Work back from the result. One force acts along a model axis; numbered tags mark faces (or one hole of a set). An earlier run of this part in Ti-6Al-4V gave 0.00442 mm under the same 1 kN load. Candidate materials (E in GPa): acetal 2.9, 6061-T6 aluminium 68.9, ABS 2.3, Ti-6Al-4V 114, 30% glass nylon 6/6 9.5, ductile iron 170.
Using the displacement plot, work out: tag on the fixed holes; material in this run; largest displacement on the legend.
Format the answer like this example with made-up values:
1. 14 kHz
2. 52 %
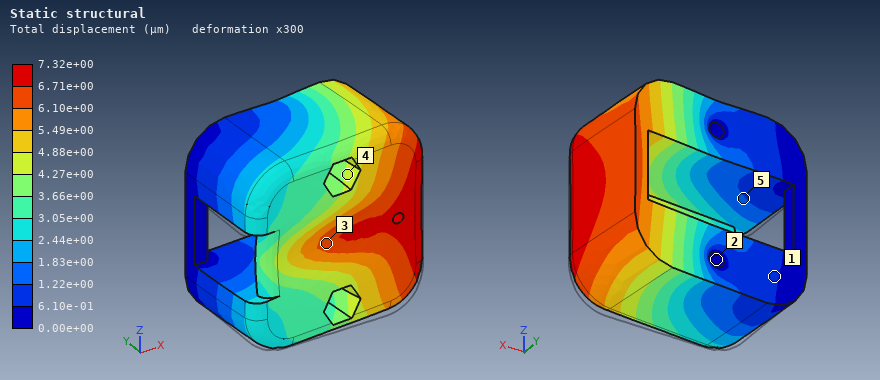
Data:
1. 2
2. 6061-T6 aluminium
3. 7.32e+00 µm
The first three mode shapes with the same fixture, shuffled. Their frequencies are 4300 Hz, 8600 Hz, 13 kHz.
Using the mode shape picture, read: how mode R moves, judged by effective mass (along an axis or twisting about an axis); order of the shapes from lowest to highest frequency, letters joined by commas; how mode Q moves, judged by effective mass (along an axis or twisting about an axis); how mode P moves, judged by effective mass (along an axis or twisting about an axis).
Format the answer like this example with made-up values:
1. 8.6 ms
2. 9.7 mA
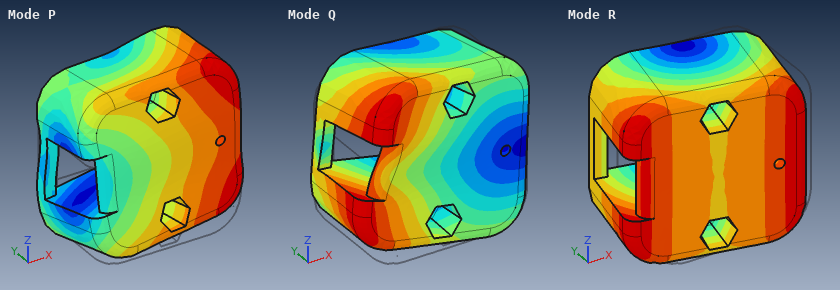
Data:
1. along X
2. R, Q, P
3. along Z
4. along Z
